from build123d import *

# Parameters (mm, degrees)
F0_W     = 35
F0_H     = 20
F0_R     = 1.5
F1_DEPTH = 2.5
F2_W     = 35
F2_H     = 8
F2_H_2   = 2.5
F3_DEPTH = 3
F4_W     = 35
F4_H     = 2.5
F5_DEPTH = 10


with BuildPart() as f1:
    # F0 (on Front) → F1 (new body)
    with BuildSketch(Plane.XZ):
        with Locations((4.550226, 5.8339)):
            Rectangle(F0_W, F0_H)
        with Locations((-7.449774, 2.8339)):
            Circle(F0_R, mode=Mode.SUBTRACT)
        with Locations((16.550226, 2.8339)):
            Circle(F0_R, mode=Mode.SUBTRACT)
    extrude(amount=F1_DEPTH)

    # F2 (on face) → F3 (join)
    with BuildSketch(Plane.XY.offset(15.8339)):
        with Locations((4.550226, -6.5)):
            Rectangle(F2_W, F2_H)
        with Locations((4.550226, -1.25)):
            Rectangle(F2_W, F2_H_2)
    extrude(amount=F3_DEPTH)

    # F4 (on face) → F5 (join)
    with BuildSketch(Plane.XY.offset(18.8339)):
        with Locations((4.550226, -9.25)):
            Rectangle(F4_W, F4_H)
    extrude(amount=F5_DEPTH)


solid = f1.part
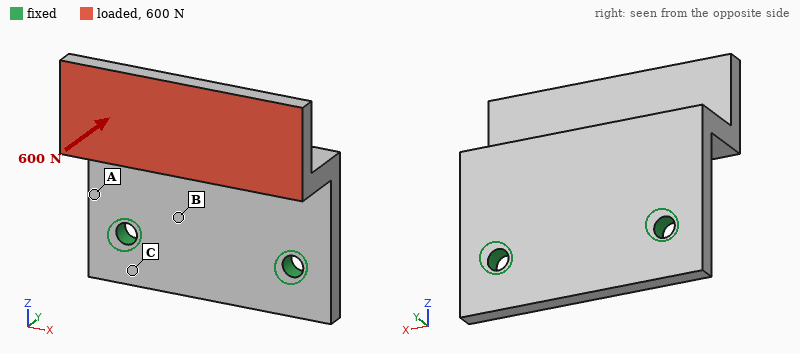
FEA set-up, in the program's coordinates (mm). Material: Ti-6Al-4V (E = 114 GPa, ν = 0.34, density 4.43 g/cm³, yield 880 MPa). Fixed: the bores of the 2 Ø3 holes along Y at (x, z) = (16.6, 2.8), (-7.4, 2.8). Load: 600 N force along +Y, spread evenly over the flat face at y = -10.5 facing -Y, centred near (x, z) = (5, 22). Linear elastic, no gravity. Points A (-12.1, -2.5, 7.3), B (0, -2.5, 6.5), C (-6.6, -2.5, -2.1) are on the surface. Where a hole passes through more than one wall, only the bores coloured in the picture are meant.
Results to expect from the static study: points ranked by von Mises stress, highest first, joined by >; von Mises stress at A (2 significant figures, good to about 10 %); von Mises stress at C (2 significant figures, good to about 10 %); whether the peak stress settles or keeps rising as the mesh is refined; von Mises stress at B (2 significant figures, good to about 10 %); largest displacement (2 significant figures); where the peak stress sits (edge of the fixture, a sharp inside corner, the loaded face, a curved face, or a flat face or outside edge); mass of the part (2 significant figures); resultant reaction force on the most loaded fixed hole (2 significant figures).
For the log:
A > B > C
270 MPa
63 MPa
keeps rising
170 MPa
0.50 mm
edge of the fixture
16 g
300 N
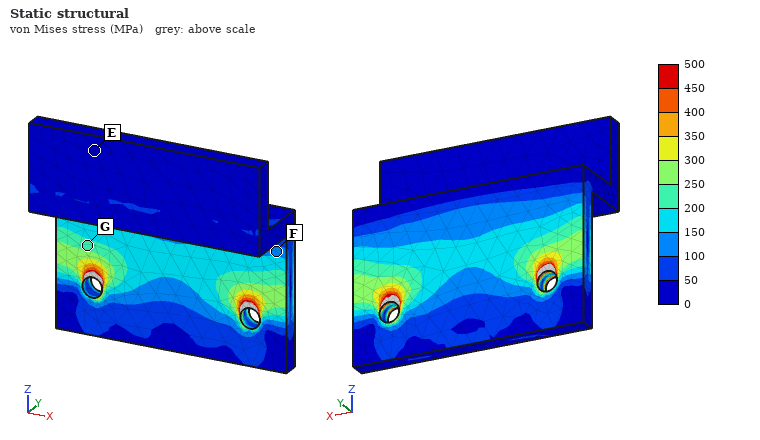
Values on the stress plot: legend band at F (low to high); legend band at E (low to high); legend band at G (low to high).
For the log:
100 to 150 MPa
0 to 50 MPa
200 to 250 MPa
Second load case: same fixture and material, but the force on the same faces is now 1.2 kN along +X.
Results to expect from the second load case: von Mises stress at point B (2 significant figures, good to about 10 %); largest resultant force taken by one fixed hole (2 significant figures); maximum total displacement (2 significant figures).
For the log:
86 MPa
1.2 kN
0.11 mm
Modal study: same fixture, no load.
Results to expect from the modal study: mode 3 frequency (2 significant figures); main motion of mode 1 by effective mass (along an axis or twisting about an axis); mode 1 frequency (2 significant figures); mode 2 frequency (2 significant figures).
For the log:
10 kHz
along Y
2300 Hz
5400 Hz
